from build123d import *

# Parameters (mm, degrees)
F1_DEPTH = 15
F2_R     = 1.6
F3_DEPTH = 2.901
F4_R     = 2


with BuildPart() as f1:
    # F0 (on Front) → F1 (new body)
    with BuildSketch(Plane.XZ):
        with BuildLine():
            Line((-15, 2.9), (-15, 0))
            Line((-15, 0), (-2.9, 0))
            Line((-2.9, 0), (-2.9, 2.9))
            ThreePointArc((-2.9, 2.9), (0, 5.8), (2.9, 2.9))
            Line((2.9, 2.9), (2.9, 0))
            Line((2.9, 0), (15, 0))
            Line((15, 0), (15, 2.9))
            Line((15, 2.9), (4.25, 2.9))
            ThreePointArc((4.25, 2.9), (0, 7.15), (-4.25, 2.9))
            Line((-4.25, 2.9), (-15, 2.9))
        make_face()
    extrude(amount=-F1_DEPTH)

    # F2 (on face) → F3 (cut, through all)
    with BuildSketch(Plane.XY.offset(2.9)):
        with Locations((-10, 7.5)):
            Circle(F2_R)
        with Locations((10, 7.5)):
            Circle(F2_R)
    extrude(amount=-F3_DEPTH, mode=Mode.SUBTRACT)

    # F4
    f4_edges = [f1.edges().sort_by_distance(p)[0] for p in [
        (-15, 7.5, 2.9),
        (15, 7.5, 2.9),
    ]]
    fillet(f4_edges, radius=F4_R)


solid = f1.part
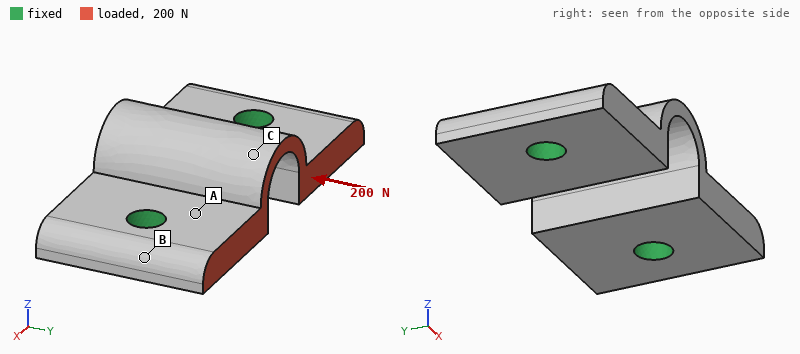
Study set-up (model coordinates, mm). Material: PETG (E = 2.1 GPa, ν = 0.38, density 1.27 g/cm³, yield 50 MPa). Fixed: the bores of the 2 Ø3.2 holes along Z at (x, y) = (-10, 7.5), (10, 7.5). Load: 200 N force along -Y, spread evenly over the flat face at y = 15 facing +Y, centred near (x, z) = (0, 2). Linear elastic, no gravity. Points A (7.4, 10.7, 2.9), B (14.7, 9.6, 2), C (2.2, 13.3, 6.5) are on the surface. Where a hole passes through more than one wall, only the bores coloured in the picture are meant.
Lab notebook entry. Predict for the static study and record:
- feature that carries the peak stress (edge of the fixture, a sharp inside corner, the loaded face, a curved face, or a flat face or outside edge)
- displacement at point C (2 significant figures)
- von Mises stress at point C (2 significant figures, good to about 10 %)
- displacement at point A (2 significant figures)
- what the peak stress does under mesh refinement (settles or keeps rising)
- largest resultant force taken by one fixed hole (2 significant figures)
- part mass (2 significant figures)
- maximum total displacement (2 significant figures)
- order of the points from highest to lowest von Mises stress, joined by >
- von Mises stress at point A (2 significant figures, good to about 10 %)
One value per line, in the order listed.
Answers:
edge of the fixture
74 µm
3.3 MPa
19 µm
keeps rising
100 N
1.5 g
89 µm
A > C > B
5.6 MPa
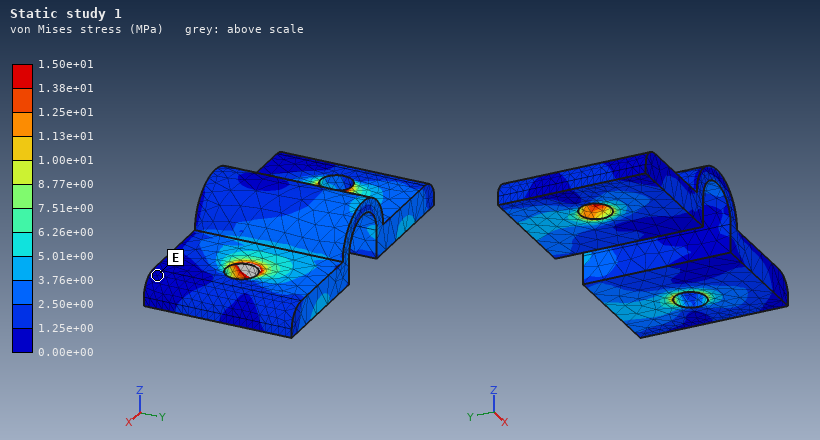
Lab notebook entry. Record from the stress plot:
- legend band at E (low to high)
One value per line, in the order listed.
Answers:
0.00e+00 to 1.25e+00 MPa
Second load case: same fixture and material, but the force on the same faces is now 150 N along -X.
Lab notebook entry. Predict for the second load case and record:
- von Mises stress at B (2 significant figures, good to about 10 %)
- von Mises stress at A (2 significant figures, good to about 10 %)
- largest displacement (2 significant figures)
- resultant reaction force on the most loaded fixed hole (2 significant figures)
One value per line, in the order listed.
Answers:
5.9 MPa
7.6 MPa
91 µm
80 N
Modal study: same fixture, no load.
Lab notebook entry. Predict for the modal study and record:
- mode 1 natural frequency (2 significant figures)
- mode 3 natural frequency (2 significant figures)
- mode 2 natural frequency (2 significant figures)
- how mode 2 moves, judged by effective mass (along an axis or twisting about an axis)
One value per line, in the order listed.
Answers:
6100 Hz
9400 Hz
8800 Hz
along Z
